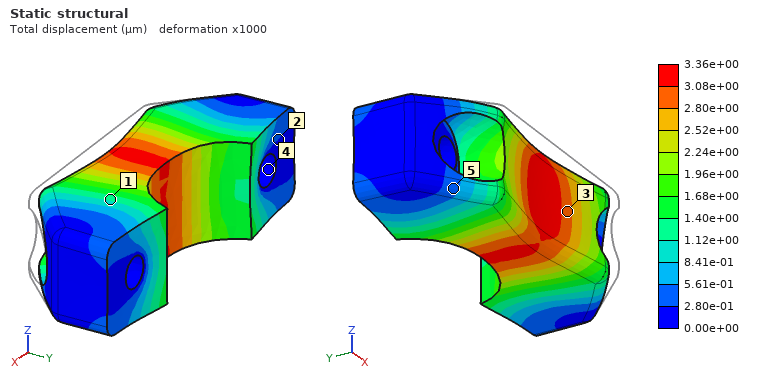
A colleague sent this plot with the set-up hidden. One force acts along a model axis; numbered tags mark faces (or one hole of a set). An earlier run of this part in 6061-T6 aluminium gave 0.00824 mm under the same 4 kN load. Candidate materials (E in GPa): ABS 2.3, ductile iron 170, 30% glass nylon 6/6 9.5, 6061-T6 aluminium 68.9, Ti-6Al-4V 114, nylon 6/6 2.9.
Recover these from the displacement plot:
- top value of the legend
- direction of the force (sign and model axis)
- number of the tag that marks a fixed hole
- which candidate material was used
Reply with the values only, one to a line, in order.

3.36e+00 µm
+Y
4
ductile iron
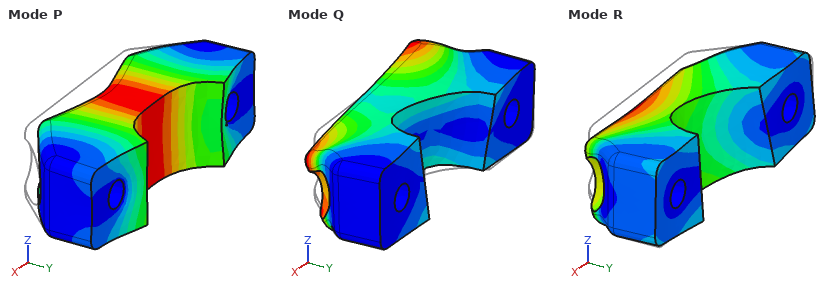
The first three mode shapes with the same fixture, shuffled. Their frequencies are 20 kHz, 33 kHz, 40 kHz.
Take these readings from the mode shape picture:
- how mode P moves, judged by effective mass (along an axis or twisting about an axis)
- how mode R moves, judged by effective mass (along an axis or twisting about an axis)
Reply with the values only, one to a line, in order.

along Y
along Z
